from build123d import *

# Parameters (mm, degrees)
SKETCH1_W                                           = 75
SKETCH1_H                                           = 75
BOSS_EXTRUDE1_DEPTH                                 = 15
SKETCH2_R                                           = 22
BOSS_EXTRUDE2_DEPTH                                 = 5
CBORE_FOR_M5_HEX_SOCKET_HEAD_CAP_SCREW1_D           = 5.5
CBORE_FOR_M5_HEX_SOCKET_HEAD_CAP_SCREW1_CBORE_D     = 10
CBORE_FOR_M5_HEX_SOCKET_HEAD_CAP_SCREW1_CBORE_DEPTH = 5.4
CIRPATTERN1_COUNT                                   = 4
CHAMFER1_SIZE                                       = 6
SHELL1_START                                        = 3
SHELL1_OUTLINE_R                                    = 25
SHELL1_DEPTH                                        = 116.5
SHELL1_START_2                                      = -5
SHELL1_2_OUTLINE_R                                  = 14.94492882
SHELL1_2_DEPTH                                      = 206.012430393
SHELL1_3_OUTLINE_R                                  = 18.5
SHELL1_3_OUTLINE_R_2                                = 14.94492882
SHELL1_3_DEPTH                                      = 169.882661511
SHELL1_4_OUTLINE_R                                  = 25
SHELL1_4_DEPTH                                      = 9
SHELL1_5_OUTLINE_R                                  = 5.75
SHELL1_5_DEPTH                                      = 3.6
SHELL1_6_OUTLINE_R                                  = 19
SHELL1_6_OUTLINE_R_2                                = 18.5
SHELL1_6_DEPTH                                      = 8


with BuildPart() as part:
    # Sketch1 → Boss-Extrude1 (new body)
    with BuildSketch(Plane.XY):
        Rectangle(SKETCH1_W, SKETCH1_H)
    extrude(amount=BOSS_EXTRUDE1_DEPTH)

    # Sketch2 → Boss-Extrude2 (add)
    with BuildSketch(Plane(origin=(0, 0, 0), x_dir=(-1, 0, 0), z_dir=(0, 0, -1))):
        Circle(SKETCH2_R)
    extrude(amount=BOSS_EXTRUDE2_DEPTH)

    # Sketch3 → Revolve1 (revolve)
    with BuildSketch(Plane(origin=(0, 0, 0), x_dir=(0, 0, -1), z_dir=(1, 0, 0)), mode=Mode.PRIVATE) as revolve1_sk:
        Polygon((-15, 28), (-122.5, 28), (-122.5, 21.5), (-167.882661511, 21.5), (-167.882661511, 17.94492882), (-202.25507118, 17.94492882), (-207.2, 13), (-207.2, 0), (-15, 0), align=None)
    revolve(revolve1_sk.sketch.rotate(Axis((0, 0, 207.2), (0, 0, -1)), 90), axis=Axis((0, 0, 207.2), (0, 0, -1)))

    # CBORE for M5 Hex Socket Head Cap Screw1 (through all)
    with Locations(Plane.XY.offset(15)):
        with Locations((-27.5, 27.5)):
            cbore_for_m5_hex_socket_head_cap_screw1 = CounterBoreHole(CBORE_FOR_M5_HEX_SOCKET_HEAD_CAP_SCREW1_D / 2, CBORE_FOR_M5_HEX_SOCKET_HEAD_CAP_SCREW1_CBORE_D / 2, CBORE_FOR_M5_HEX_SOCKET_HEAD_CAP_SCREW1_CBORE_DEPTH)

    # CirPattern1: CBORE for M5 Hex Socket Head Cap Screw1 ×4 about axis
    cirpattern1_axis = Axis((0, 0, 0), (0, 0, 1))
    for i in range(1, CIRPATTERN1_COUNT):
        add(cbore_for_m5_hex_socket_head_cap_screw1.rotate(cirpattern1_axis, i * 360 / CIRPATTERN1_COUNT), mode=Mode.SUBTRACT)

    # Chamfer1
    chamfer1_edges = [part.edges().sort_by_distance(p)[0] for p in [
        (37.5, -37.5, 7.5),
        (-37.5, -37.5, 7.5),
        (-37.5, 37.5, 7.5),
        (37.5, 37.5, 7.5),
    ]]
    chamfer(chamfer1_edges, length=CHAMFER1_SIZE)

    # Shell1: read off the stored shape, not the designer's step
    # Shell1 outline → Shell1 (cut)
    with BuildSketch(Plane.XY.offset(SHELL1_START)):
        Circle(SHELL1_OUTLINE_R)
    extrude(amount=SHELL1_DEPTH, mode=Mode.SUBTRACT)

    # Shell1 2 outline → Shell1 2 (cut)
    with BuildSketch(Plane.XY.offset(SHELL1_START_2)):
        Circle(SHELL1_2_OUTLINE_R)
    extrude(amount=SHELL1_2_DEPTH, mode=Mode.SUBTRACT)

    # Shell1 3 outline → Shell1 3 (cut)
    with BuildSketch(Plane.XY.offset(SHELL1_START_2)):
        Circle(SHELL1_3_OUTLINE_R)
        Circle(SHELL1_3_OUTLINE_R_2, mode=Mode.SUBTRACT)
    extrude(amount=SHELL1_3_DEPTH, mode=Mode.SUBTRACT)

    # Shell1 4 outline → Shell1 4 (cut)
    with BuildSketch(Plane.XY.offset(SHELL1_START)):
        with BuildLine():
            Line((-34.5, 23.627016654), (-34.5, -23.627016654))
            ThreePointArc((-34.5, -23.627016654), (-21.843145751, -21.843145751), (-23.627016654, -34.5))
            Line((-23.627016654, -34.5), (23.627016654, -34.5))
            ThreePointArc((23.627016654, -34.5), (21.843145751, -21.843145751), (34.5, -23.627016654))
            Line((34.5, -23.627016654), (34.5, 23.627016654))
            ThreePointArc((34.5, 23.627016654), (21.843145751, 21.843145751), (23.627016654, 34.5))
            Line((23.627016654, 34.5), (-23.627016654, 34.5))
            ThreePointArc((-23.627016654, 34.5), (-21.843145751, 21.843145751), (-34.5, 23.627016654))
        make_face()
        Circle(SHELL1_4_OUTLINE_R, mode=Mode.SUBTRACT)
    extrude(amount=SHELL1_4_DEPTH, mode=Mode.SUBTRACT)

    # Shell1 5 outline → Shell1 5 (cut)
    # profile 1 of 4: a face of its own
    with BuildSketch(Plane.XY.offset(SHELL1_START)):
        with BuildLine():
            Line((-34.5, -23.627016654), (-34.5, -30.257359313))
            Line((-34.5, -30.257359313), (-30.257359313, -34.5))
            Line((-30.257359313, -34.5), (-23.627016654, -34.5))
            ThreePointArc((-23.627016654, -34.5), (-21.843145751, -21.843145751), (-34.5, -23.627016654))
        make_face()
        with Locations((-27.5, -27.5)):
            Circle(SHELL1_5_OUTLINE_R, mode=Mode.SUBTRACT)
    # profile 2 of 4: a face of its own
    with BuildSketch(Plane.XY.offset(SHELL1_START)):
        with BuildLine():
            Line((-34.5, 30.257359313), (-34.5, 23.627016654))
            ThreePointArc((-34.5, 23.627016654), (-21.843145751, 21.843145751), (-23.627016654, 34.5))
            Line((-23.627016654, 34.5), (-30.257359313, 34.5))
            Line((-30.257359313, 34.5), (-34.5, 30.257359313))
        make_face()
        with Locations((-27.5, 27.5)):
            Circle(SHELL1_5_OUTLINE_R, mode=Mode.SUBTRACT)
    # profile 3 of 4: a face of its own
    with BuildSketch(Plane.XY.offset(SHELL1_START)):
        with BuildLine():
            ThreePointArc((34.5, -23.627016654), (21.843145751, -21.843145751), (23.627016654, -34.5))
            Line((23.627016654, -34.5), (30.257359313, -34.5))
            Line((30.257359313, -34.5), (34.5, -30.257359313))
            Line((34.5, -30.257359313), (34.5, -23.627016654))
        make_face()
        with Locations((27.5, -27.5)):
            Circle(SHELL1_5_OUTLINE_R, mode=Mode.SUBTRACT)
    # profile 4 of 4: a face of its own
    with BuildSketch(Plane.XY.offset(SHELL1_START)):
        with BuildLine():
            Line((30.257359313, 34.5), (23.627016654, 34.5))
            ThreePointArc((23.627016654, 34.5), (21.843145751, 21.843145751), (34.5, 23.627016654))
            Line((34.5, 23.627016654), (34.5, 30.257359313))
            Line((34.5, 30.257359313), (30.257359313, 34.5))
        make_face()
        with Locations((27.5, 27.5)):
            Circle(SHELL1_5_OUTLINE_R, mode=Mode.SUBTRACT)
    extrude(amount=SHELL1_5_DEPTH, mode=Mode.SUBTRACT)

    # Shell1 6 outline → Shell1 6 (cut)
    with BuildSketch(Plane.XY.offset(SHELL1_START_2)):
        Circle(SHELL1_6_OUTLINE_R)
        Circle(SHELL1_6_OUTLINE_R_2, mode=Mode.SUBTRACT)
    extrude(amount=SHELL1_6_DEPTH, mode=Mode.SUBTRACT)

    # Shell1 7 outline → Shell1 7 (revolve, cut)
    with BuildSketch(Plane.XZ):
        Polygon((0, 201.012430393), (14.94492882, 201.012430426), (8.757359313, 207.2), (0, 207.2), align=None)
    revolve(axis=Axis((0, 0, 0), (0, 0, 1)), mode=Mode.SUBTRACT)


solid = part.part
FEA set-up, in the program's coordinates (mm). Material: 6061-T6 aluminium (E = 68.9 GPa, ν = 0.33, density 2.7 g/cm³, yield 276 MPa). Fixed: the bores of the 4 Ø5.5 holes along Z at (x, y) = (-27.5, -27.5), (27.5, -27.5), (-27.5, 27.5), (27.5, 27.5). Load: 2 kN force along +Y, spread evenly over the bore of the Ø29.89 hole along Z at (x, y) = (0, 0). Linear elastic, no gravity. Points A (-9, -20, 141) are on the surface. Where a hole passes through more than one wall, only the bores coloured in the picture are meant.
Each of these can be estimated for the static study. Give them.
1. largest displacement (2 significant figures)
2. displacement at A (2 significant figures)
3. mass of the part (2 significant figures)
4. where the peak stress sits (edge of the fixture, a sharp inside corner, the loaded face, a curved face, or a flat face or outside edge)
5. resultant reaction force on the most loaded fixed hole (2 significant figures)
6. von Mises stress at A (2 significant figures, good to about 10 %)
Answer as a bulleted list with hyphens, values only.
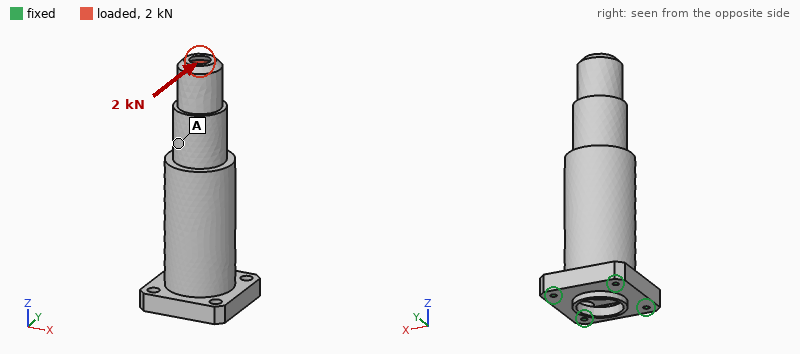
- 1.1 mm
- 0.63 mm
- 330 g
- a flat face or outside edge
- 3.9 kN
- 18 MPa
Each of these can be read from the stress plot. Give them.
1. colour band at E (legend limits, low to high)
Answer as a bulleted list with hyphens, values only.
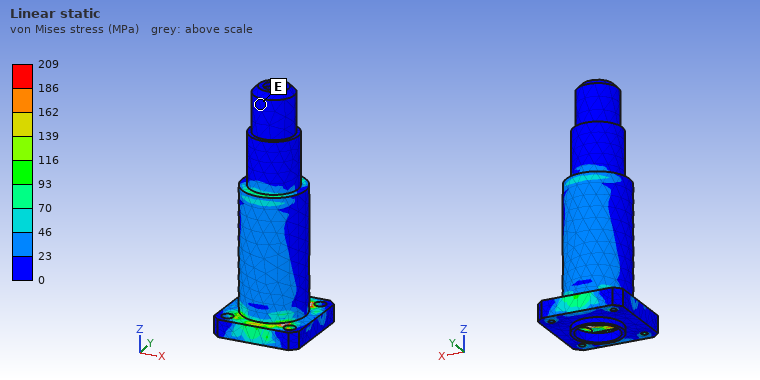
- 0 to 23 MPa
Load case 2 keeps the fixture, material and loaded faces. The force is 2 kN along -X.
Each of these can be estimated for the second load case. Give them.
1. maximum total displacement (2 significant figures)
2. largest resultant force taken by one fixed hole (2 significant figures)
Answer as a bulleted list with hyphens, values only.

- 1.1 mm
- 3.9 kN
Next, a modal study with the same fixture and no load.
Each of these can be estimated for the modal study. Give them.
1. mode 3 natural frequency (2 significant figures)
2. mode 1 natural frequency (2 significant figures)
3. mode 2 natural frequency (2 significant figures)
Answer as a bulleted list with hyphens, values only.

- 3900 Hz
- 820 Hz
- 830 Hz
